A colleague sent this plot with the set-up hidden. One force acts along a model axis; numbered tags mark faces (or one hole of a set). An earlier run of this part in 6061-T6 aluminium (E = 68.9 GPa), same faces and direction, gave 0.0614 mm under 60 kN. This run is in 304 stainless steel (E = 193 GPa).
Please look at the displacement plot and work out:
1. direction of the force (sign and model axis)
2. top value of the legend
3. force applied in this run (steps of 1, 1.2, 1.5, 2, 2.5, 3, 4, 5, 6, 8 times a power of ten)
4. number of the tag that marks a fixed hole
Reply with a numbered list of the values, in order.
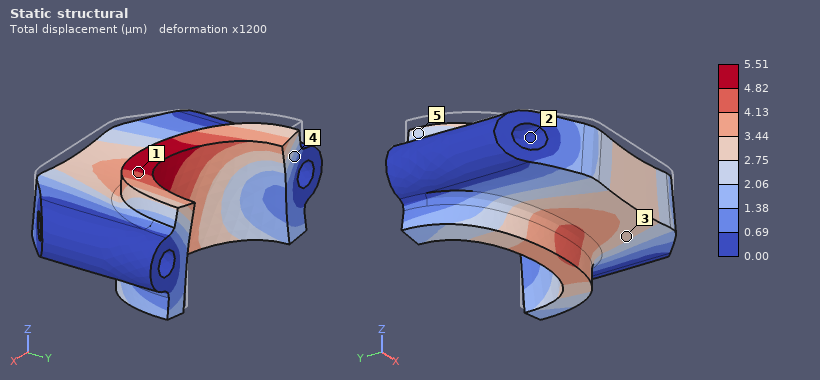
1. -Z
2. 5.51 µm
3. 15 kN
4. 2
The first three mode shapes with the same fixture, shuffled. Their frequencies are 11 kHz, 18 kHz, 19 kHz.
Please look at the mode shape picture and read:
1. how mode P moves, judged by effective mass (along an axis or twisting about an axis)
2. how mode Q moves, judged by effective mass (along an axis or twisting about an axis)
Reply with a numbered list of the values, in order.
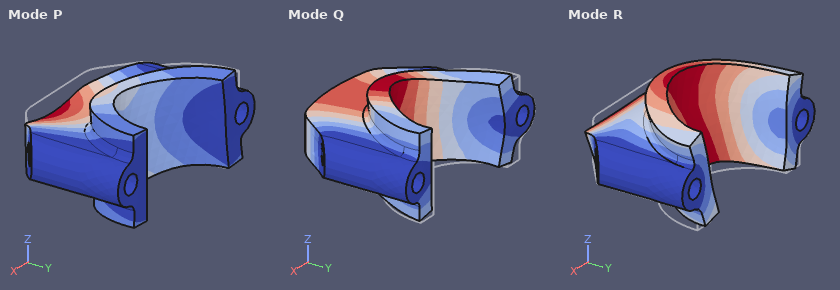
1. along Z
2. along Y
